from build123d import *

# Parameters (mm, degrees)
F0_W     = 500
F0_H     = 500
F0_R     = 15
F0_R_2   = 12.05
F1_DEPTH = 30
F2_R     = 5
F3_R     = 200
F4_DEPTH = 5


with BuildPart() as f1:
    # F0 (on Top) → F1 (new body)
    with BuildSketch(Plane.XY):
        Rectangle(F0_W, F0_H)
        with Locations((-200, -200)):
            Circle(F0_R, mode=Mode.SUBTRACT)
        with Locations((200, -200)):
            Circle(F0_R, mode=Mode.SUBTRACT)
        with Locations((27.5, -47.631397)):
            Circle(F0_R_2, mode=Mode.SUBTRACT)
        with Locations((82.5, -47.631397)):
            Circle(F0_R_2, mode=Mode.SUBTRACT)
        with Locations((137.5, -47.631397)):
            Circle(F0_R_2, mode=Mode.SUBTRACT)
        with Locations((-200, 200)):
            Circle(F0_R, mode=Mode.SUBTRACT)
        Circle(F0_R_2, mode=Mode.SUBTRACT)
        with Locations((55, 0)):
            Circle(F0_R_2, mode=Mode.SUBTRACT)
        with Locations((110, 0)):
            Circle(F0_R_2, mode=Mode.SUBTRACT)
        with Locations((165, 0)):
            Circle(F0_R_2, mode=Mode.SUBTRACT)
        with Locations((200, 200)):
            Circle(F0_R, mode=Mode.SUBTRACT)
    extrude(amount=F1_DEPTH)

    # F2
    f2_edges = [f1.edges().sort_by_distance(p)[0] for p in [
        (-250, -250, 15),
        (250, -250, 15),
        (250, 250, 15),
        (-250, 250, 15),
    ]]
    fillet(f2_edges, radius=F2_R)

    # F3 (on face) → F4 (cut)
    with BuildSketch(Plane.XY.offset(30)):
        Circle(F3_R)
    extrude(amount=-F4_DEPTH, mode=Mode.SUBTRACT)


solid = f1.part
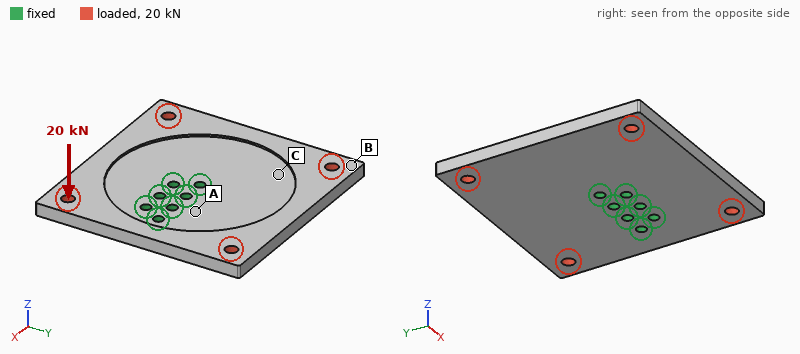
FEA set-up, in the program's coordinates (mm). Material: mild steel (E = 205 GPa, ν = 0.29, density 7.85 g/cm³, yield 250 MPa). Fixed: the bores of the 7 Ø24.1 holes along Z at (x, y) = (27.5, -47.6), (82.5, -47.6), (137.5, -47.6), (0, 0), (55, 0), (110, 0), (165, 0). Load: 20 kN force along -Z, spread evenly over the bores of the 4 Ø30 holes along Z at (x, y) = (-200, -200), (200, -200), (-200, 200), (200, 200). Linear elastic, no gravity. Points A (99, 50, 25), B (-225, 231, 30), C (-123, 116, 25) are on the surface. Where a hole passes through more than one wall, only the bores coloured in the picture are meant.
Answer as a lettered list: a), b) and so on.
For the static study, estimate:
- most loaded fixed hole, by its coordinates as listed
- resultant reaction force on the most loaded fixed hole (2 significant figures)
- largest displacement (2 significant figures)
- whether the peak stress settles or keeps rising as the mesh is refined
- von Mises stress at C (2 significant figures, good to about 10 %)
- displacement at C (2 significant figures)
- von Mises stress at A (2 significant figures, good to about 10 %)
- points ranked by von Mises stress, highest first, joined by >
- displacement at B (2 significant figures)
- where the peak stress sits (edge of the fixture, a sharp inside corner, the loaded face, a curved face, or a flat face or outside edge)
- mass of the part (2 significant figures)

a) (0, 0)
b) 15 kN
c) 0.52 mm
d) keeps rising
e) 12 MPa
f) 0.19 mm
g) 22 MPa
h) A > C > B
i) 0.46 mm
j) edge of the fixture
k) 53 kg
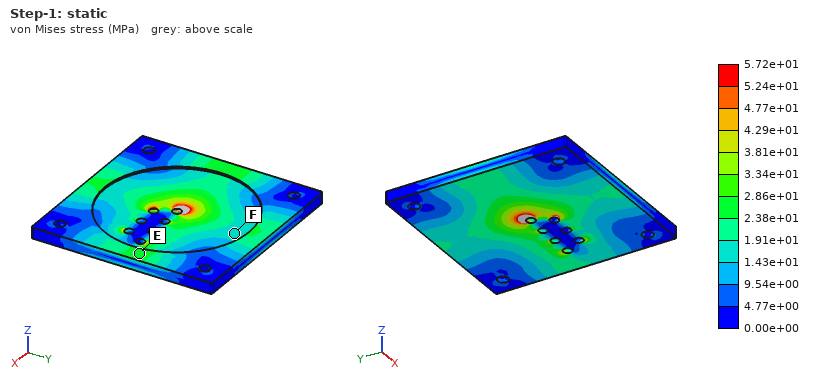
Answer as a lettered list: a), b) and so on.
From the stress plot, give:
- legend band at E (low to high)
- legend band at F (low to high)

a) 2.38e+01 to 2.86e+01 MPa
b) 1.43e+01 to 1.91e+01 MPa
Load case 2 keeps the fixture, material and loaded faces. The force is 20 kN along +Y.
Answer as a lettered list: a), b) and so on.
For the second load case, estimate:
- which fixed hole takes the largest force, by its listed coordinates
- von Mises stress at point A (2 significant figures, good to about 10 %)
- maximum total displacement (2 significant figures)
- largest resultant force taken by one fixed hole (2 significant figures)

a) (0, 0)
b) 2.2 MPa
c) 13 µm
d) 11 kN
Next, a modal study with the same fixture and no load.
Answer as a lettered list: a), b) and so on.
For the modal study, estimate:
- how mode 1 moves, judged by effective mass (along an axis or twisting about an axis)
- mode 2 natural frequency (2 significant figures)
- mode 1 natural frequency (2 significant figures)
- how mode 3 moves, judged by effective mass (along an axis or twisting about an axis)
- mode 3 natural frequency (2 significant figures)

a) along Z
b) 260 Hz
c) 240 Hz
d) along Z
e) 410 Hz
